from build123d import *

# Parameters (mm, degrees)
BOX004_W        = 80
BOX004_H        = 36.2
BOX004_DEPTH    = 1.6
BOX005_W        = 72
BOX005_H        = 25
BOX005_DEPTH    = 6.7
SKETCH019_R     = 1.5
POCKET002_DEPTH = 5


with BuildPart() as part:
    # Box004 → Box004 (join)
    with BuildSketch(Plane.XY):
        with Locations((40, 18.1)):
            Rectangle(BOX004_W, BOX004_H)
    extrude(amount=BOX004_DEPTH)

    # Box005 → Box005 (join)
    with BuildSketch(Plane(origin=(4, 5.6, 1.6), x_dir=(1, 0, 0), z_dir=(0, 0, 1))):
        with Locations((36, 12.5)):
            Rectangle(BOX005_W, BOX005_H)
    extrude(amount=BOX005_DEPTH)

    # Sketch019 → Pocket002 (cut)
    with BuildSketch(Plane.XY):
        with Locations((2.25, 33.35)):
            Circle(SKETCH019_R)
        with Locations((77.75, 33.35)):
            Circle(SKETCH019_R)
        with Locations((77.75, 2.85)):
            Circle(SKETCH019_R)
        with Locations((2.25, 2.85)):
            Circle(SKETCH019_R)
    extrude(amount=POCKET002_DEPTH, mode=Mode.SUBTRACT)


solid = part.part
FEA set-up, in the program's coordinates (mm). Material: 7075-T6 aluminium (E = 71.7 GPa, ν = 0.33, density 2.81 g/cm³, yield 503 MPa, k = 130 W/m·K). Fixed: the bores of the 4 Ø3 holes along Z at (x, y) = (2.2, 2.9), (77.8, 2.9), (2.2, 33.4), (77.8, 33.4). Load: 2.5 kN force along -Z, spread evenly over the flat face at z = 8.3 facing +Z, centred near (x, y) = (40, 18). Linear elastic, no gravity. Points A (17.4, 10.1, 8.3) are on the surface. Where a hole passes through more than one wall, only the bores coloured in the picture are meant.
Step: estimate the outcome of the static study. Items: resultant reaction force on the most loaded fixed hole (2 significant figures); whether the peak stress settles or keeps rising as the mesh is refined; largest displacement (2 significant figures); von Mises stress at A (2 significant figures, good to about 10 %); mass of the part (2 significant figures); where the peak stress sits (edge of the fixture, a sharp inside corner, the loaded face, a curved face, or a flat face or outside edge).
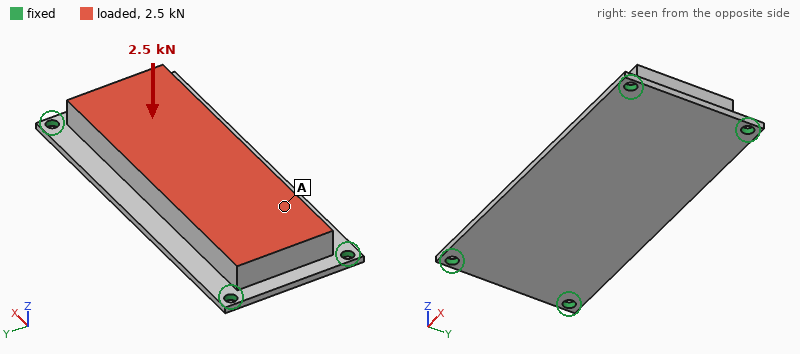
1.2 kN
keeps rising
0.12 mm
34 MPa
47 g
edge of the fixture
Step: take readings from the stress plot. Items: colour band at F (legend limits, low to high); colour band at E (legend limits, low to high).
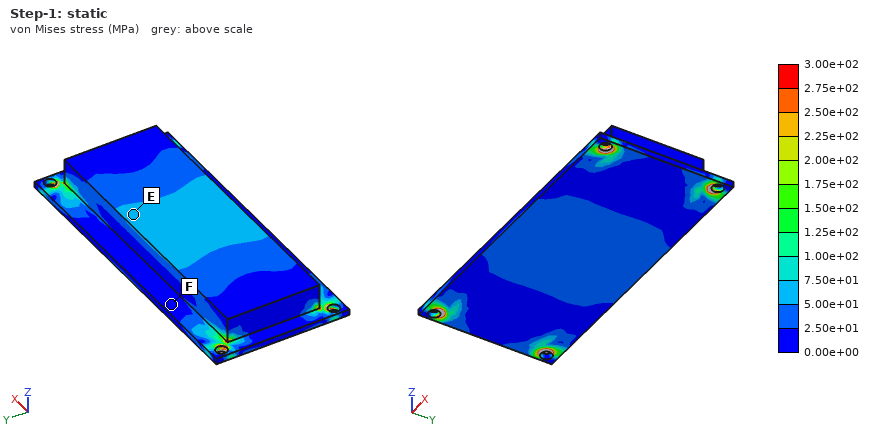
0.00e+00 to 2.50e+01 MPa
5.00e+01 to 7.50e+01 MPa
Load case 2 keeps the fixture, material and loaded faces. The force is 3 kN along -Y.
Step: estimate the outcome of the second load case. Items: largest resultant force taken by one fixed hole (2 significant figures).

1.0 kN
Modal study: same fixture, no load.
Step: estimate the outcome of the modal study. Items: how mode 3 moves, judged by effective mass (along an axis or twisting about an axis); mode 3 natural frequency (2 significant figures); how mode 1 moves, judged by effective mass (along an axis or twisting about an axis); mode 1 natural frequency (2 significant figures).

twisting about Y
9200 Hz
along Z
3800 Hz
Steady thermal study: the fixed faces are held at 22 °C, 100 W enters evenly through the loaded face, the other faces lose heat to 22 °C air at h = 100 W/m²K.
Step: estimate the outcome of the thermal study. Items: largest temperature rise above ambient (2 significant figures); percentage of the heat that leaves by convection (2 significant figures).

70 K
30 %
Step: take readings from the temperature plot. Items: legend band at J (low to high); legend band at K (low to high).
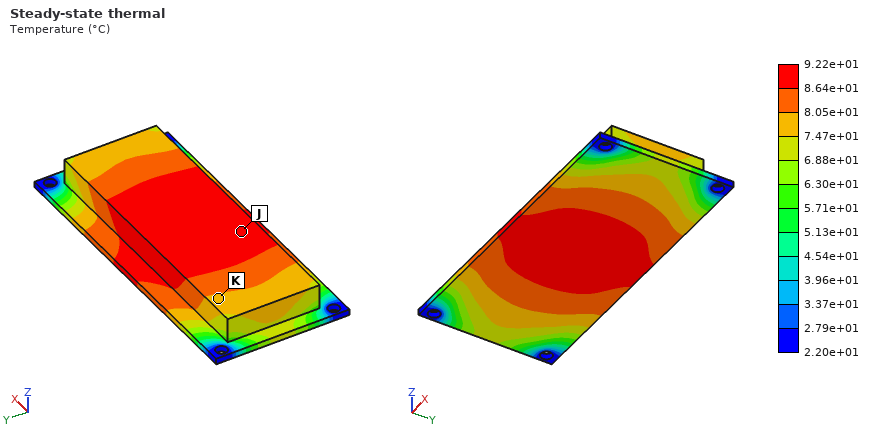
8.64e+01 to 9.22e+01 °C
7.47e+01 to 8.05e+01 °C
